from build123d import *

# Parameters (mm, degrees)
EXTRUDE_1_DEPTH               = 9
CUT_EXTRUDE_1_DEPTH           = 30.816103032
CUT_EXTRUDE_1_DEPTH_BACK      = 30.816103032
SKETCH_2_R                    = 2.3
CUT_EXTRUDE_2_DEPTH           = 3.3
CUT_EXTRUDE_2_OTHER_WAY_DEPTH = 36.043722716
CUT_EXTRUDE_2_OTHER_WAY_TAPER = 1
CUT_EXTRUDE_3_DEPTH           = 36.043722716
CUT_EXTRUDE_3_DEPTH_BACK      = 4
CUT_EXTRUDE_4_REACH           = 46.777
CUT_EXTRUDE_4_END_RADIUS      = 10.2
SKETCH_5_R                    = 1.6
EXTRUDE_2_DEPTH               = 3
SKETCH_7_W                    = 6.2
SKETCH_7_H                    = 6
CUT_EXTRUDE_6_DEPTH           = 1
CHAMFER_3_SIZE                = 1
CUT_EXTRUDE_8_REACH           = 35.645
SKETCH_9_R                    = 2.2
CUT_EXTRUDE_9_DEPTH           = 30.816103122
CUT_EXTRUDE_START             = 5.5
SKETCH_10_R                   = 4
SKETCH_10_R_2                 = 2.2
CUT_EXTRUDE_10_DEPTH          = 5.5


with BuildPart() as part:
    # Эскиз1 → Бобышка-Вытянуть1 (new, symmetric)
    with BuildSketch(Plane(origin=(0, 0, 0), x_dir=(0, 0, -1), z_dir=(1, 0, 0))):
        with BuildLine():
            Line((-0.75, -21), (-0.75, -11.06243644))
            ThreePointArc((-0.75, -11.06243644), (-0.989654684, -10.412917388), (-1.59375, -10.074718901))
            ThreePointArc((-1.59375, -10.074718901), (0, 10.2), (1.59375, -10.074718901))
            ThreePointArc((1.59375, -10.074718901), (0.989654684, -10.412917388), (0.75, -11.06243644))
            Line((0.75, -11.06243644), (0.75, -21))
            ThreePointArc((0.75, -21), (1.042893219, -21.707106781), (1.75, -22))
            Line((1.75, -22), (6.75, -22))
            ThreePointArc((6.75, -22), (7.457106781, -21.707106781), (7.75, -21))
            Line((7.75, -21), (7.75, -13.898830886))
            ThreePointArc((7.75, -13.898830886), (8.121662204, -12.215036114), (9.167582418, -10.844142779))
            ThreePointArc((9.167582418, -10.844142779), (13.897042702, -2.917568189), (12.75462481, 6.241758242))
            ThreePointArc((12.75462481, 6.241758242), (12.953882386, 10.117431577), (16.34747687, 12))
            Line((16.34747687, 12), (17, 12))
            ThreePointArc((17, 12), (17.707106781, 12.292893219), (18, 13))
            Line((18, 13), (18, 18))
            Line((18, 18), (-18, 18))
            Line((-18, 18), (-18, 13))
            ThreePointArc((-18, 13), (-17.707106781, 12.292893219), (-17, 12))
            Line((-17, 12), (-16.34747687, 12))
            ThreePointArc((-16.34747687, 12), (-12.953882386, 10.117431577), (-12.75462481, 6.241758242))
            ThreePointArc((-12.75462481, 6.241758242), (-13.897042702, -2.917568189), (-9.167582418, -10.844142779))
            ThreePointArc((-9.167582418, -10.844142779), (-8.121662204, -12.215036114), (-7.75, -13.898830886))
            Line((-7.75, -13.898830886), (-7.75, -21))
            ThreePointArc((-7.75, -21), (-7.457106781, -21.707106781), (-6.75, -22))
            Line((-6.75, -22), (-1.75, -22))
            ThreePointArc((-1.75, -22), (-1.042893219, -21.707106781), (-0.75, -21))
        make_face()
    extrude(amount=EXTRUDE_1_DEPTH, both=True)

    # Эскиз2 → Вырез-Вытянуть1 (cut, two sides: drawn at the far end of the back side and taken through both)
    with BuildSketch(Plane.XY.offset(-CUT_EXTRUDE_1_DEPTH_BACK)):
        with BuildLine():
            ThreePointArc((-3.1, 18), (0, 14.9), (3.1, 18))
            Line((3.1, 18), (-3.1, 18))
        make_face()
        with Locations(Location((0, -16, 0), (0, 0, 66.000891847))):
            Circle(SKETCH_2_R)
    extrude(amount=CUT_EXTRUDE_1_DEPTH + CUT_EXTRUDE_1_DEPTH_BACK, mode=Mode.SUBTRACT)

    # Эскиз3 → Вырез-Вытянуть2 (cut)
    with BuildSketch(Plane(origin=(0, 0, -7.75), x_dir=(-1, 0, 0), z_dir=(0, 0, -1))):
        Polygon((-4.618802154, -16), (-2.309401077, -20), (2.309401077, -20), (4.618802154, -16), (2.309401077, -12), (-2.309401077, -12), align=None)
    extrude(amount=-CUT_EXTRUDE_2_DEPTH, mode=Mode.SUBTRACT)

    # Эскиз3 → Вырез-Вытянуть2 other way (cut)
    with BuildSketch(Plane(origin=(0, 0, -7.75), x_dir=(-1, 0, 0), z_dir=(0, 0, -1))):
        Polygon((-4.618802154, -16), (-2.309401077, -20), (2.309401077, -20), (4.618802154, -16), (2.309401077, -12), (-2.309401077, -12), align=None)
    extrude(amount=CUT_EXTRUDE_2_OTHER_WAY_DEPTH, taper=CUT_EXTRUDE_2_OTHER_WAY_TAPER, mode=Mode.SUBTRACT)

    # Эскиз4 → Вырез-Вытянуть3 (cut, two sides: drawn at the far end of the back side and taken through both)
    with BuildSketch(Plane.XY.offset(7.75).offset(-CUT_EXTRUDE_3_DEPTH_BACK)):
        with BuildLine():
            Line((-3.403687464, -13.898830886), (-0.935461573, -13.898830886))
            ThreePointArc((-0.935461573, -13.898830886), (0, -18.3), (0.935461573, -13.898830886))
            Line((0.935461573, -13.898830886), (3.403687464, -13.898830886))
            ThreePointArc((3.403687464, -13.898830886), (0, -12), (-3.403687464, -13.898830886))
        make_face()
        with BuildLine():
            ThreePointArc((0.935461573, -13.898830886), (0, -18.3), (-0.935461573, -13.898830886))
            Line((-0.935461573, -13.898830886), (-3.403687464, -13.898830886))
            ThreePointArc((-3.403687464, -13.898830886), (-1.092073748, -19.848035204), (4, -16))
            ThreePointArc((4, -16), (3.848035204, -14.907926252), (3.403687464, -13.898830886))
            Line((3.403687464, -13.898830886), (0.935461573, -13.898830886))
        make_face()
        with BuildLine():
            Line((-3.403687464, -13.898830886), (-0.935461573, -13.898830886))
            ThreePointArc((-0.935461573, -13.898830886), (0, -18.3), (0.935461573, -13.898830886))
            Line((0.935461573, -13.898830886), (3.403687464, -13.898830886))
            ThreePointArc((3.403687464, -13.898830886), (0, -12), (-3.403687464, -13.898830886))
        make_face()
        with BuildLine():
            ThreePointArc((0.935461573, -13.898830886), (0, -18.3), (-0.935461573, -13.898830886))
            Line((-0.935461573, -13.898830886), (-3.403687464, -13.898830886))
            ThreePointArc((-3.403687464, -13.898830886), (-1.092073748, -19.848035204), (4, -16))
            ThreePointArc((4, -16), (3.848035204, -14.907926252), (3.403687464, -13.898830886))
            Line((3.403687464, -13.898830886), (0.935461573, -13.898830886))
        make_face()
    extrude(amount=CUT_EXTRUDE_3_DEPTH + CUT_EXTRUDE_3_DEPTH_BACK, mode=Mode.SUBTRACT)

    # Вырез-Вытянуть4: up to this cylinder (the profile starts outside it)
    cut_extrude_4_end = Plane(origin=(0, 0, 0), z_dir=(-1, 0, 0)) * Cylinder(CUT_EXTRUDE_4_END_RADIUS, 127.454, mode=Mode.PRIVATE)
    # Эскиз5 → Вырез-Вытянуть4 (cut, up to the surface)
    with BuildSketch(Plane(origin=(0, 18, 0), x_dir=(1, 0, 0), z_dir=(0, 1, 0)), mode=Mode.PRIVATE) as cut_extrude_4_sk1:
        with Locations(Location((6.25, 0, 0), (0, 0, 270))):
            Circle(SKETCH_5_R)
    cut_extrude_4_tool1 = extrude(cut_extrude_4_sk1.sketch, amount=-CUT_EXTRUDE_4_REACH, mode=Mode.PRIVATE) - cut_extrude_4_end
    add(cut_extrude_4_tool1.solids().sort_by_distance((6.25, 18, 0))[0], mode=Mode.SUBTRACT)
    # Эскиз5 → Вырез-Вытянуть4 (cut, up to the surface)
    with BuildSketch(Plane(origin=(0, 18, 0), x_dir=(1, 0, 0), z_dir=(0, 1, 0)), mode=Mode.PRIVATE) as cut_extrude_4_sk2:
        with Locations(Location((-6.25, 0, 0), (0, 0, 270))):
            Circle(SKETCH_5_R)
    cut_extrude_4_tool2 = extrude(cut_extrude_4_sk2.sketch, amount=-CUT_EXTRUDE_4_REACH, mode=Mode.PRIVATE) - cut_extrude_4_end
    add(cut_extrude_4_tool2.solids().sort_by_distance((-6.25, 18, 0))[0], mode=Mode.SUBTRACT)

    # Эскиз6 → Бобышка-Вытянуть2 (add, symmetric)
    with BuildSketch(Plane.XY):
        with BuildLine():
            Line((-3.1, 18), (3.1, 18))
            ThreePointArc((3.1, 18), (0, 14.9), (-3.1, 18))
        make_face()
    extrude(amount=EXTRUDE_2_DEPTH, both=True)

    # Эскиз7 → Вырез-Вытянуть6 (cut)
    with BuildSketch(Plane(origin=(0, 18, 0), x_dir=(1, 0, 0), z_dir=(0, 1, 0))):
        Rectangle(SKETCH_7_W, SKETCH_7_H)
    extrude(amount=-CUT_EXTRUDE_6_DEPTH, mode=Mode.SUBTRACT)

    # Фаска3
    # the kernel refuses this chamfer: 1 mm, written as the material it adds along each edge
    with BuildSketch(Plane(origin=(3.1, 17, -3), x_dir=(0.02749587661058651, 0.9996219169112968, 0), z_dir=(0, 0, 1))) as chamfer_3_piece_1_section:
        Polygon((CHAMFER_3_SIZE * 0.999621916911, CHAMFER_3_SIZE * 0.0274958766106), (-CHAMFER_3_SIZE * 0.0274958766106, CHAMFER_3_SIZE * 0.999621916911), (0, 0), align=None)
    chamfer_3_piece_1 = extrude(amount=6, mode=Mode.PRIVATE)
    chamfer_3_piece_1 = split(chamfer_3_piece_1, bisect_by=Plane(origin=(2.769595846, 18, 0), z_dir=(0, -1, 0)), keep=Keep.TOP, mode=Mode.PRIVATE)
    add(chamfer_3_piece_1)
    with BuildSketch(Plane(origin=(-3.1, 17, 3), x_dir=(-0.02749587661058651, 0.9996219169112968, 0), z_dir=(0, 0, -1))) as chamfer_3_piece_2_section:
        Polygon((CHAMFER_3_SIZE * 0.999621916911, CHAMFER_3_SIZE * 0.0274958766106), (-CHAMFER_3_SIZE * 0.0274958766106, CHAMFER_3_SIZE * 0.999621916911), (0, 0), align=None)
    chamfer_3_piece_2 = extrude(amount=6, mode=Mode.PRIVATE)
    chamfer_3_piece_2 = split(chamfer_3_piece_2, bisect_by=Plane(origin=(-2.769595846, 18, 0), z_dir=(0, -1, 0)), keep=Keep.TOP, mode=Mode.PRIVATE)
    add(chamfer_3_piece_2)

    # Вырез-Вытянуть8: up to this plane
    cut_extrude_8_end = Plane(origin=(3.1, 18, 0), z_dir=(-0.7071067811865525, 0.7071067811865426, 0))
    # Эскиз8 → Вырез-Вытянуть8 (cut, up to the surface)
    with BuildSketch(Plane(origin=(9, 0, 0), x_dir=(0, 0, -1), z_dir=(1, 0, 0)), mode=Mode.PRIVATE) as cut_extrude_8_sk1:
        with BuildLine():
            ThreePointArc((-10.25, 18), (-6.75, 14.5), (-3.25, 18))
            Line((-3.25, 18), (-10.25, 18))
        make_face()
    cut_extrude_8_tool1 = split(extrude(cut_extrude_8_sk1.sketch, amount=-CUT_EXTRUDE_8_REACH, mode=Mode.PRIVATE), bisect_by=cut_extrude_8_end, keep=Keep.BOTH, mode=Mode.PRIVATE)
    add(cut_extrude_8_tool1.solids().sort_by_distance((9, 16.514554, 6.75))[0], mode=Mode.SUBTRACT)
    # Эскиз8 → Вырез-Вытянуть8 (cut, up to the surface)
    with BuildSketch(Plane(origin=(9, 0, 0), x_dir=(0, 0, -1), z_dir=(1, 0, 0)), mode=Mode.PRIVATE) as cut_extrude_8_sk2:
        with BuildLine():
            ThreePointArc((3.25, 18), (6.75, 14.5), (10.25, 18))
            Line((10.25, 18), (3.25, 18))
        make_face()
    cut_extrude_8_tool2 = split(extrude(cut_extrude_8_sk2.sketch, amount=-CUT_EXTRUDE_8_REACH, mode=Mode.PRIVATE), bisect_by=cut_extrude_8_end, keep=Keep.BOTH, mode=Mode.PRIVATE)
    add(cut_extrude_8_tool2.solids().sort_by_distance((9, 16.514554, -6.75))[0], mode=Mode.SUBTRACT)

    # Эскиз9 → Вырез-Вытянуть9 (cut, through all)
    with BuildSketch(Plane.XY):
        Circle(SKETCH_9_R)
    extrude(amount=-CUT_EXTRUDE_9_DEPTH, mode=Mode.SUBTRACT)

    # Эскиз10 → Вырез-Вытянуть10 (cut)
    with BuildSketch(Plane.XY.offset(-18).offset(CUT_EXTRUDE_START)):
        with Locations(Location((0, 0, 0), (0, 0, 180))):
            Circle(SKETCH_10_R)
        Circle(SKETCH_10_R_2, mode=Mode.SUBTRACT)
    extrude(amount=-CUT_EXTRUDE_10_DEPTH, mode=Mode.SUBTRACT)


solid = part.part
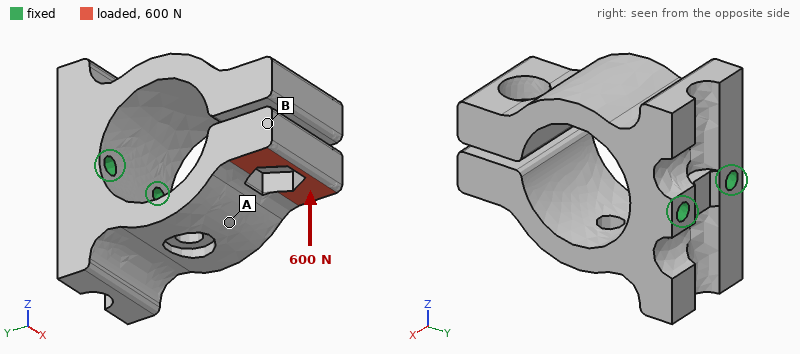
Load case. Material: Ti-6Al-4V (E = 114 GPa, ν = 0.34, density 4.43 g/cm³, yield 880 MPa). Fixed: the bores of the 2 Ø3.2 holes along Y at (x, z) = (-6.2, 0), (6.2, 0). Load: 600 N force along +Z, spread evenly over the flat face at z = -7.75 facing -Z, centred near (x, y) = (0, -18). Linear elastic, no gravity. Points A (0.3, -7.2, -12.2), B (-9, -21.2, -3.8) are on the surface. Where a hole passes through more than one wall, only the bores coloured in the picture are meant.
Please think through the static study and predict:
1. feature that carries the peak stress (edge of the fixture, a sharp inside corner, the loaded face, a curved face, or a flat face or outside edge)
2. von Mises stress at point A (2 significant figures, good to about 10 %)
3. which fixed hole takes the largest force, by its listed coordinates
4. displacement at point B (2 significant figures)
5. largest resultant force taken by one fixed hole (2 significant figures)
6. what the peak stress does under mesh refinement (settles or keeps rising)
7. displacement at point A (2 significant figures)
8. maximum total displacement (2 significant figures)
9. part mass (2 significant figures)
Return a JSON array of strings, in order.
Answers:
["a sharp inside corner", "79 MPa", "(6.2, 0)", "0.59 mm", "380 N", "keeps rising", "0.23 mm", "0.63 mm", "45 g"]
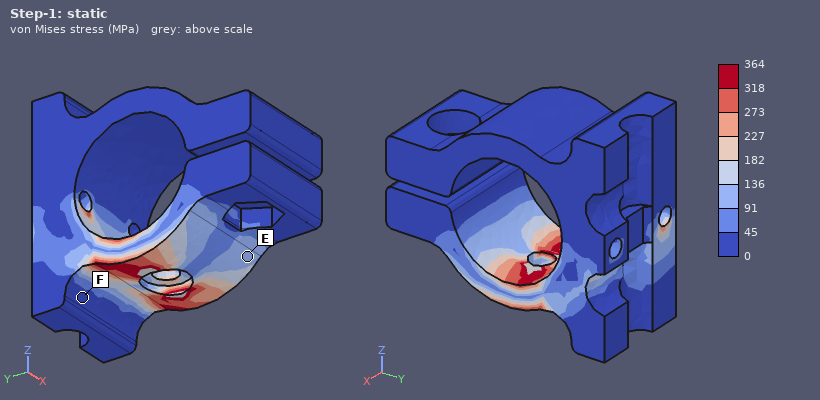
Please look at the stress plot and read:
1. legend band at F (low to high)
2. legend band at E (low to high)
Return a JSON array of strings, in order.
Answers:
["0 to 45 MPa", "91 to 136 MPa"]
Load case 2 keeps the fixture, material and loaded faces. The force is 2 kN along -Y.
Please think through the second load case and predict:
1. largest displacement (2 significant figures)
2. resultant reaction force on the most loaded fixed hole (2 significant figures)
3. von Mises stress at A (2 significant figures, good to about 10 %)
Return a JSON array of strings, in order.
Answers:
["0.28 mm", "1.0 kN", "50 MPa"]
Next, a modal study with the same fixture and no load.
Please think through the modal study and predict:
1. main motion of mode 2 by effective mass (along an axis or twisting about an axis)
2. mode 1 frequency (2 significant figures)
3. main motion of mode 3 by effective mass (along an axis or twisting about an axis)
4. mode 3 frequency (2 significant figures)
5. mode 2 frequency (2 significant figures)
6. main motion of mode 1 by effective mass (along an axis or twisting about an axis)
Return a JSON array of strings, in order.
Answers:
["along Z", "2300 Hz", "along X", "4400 Hz", "2500 Hz", "along Z"]
